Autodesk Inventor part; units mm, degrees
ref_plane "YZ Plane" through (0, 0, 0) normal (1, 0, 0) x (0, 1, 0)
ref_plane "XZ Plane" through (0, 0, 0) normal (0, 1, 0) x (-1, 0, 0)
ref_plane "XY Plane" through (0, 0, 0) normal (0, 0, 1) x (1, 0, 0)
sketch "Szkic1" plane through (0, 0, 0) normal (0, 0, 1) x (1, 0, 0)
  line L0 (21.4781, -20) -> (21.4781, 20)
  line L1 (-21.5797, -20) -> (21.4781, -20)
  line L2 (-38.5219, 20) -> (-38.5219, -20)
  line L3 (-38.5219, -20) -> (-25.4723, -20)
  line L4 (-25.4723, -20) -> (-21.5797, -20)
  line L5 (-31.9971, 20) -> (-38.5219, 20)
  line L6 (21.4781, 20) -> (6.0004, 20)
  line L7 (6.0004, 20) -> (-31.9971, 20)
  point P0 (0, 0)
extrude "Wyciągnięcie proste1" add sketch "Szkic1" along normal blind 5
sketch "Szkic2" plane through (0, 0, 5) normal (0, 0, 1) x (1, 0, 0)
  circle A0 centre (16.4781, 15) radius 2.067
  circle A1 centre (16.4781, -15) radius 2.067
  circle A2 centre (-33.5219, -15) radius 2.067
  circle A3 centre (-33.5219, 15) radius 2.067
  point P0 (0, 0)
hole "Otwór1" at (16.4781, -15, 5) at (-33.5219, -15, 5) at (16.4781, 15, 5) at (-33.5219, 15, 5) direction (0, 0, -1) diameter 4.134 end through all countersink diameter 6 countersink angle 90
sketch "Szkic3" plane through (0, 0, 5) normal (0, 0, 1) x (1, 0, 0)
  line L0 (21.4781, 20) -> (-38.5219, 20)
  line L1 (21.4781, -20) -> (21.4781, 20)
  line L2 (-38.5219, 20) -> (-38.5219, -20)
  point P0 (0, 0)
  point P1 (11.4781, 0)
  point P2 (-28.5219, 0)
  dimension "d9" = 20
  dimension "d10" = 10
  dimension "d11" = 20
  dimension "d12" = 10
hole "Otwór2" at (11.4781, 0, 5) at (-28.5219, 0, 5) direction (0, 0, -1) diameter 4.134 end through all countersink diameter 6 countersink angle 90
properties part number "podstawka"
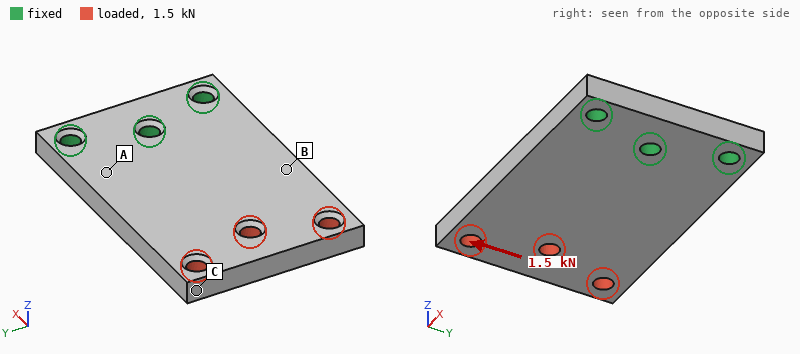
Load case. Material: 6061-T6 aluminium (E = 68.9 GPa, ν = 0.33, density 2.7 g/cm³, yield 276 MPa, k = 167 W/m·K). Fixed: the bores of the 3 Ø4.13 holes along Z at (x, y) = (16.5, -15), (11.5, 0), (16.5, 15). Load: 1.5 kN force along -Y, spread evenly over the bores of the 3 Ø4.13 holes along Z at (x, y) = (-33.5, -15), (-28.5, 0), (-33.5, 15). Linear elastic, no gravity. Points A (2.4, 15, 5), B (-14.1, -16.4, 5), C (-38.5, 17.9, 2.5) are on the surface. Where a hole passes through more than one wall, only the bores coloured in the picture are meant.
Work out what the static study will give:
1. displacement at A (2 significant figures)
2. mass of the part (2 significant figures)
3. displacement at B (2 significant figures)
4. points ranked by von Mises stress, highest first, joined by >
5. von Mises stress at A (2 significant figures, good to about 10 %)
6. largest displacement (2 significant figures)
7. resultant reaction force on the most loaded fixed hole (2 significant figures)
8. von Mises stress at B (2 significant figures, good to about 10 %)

11 µm
31 g
28 µm
A > B > C
30 MPa
62 µm
2.1 kN
17 MPa
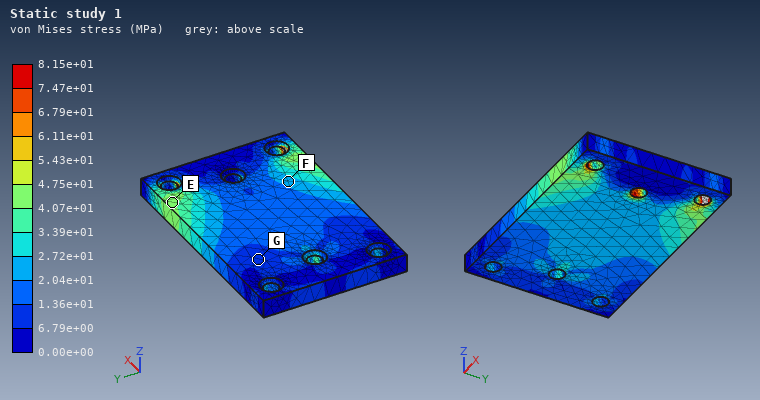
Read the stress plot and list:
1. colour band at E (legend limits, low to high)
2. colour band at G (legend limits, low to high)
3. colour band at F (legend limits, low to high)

4.07e+01 to 4.75e+01 MPa
6.79e+00 to 1.36e+01 MPa
2.04e+01 to 2.72e+01 MPa
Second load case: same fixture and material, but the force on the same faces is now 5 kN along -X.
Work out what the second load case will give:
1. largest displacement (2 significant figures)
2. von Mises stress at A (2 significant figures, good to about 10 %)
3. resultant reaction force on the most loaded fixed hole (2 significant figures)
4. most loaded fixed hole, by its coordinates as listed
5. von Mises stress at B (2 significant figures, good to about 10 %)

0.10 mm
11 MPa
2.1 kN
(11.5, 0)
11 MPa
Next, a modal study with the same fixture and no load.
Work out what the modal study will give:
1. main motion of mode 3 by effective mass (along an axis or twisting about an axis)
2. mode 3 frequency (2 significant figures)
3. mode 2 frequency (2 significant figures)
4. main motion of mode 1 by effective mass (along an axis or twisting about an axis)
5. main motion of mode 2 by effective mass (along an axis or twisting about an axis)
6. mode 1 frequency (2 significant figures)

along Y
8400 Hz
4200 Hz
along Z
twisting about X
1600 Hz
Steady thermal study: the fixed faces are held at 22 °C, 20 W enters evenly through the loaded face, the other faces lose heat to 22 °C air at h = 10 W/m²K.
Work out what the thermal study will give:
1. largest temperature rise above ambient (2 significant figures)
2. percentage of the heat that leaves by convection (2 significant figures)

30 K
3.8 %
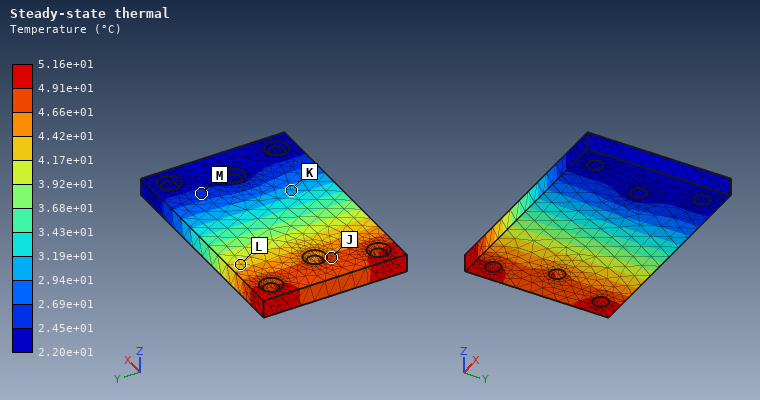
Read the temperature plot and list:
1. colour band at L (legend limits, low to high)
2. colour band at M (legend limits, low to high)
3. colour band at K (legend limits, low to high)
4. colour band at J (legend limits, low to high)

4.17e+01 to 4.42e+01 °C
2.45e+01 to 2.69e+01 °C
2.94e+01 to 3.19e+01 °C
4.66e+01 to 4.91e+01 °C
